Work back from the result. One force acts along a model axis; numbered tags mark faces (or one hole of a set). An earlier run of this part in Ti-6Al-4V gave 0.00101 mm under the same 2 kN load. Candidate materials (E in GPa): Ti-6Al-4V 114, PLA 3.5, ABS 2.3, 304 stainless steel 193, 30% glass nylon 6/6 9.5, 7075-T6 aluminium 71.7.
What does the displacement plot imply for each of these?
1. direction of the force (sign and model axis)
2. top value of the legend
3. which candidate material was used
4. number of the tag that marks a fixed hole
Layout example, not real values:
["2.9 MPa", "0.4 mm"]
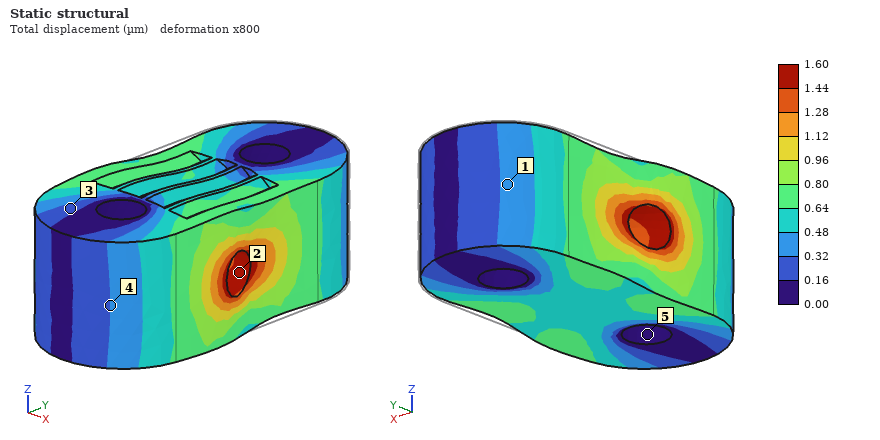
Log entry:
["-Y", "1.60 µm", "7075-T6 aluminium", "5"]
